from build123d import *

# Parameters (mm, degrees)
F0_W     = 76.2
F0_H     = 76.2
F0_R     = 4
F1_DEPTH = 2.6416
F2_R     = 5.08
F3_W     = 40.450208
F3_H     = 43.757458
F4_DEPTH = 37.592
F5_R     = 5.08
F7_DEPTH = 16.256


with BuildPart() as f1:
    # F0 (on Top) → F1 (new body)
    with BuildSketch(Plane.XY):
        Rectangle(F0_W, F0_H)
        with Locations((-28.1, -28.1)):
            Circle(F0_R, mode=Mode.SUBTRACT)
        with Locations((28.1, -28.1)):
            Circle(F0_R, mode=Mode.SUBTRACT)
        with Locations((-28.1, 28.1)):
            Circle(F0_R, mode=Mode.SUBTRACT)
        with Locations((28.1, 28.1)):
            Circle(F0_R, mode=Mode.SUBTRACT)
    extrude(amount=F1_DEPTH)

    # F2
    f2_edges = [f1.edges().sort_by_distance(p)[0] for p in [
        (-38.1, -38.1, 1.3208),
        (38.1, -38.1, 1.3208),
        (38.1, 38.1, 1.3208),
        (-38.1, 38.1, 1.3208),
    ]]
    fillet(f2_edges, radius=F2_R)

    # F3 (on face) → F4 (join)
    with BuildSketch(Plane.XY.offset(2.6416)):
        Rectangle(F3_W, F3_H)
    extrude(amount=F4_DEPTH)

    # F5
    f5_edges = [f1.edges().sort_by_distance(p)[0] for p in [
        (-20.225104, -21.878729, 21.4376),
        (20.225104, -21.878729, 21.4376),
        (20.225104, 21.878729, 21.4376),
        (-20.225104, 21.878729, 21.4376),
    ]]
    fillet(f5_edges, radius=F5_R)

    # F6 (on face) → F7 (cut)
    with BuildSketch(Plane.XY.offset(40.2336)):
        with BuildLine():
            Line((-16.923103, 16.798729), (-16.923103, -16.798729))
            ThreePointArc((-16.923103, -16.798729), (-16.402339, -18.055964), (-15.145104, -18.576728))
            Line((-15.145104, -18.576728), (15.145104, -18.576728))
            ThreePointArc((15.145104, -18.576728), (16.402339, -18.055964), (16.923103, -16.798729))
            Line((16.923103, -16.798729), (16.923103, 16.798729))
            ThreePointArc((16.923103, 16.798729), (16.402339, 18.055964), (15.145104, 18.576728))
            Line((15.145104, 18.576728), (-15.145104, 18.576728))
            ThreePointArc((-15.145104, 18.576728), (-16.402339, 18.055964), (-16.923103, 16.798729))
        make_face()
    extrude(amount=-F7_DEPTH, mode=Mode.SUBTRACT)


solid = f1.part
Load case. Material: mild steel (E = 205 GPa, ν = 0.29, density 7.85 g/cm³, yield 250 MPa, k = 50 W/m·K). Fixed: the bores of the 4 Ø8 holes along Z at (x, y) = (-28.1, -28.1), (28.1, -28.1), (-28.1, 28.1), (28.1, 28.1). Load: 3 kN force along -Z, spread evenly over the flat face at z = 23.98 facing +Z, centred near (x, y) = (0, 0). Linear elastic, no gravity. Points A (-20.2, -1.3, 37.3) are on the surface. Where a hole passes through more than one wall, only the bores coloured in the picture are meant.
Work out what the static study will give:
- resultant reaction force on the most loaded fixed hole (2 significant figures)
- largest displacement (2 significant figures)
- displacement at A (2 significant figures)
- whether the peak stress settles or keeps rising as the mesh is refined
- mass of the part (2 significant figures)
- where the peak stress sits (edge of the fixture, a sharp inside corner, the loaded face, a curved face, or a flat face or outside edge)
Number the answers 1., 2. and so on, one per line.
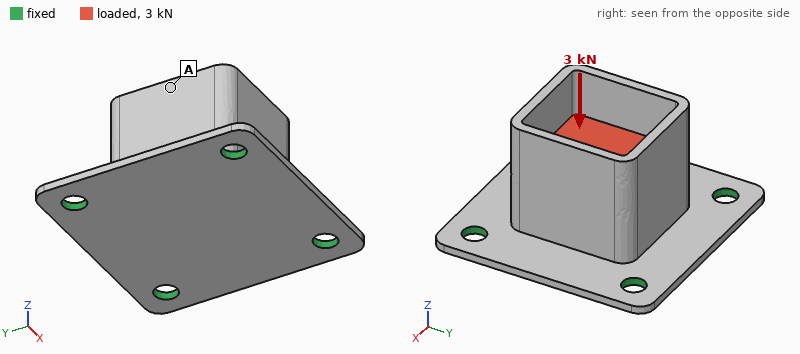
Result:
1. 840 N
2. 19 µm
3. 19 µm
4. keeps rising
5. 470 g
6. edge of the fixture
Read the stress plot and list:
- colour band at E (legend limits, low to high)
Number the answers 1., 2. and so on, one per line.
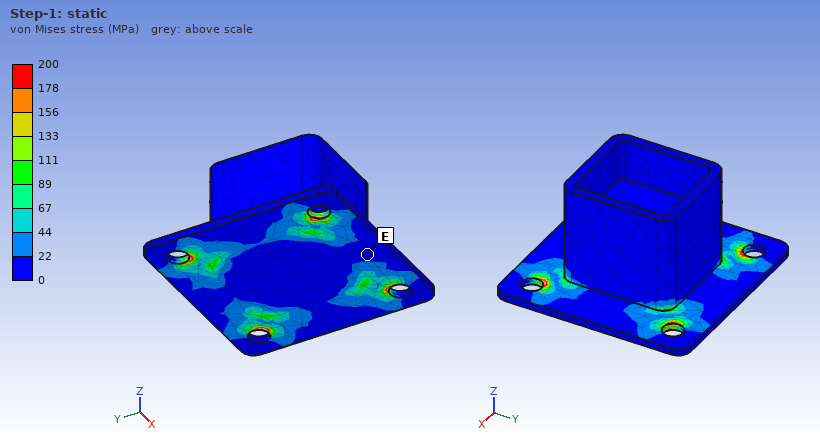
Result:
1. 0 to 22 MPa
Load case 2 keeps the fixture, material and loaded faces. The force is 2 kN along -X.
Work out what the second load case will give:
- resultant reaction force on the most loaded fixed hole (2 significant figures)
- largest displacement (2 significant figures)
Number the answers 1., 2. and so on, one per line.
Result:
1. 750 N
2. 25 µm
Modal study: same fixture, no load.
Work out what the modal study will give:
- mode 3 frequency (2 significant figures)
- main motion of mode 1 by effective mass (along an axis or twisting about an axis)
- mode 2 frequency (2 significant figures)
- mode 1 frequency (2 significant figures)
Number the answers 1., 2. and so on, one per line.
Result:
1. 3300 Hz
2. along Z
3. 3300 Hz
4. 3100 Hz
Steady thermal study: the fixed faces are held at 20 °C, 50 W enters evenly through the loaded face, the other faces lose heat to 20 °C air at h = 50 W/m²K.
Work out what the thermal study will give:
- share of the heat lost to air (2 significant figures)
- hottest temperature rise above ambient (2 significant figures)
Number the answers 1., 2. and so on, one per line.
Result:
1. 47 %
2. 44 K
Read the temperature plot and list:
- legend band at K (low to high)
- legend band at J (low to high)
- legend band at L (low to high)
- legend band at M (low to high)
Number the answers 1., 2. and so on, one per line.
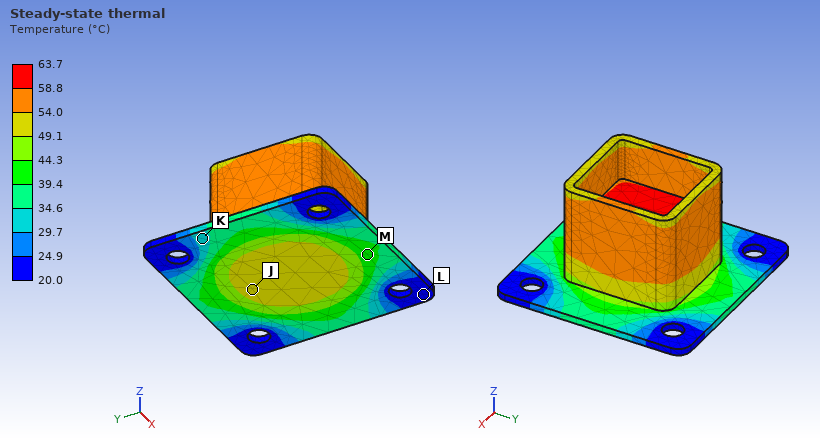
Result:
1. 29.7 to 34.6 °C
2. 49.1 to 54.0 °C
3. 20.0 to 24.9 °C
4. 39.4 to 44.3 °C
